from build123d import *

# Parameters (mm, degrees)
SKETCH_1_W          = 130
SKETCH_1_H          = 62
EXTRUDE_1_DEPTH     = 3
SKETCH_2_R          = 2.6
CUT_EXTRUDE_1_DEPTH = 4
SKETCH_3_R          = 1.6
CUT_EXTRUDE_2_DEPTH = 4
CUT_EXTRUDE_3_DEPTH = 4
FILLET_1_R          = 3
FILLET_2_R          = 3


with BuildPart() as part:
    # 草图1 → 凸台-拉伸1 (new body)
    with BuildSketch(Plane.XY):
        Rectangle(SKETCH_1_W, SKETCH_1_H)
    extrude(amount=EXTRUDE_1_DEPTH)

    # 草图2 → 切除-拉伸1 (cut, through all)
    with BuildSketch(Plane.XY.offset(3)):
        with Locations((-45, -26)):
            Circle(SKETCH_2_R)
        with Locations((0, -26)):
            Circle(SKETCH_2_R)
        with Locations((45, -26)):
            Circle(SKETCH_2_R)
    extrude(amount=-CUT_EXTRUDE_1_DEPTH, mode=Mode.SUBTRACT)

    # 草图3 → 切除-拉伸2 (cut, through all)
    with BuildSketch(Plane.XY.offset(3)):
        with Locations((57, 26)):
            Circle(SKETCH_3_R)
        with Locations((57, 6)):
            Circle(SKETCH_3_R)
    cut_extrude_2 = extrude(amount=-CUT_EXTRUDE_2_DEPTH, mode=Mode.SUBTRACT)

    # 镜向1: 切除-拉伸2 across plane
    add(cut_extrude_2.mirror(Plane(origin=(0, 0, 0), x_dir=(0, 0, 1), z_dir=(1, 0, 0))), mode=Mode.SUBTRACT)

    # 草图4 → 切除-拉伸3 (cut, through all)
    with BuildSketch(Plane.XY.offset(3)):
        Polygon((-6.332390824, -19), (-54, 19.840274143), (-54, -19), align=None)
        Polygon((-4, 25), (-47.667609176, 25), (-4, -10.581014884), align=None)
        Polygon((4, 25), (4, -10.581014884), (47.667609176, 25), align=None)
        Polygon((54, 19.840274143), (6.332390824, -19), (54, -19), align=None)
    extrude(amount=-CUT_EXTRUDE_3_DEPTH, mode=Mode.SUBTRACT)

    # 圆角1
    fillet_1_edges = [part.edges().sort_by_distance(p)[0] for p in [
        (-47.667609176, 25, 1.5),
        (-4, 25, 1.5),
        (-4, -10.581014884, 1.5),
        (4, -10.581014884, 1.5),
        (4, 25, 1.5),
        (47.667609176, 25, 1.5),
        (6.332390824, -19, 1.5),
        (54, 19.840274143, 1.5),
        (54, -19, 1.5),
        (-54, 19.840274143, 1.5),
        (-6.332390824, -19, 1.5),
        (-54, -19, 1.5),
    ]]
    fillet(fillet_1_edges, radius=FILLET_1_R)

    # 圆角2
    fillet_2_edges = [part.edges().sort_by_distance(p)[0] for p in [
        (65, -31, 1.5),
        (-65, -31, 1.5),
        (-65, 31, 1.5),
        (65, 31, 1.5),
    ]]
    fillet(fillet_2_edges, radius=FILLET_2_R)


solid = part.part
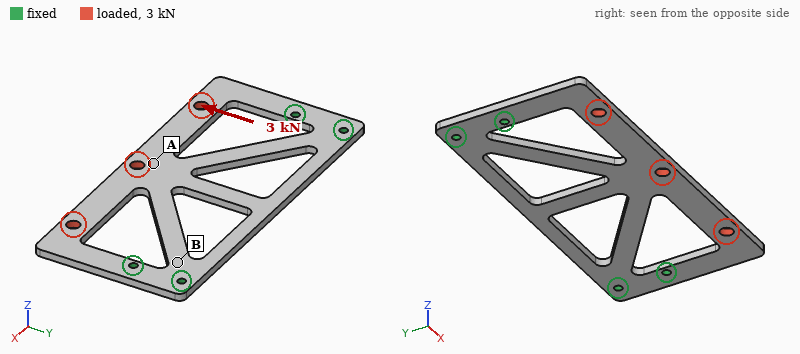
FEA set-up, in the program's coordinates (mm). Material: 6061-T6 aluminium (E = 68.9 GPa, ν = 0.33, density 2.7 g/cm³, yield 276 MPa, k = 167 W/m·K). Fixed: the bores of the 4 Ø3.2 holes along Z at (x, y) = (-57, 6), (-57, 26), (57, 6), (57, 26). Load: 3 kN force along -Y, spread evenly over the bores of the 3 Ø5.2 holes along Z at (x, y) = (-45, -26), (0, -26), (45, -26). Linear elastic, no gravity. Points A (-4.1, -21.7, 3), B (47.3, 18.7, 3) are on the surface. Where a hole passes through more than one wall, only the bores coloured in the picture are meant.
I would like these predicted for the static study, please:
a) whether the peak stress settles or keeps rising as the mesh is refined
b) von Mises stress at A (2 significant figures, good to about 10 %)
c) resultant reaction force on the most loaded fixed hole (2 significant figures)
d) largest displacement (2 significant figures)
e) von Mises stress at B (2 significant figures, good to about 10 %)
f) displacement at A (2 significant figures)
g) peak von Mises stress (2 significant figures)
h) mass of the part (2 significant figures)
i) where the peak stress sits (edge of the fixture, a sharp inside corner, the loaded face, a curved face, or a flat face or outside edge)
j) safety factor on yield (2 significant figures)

settles
20 MPa
1.0 kN
70 µm
36 MPa
63 µm
180 MPa
38 g
a curved face
1.6
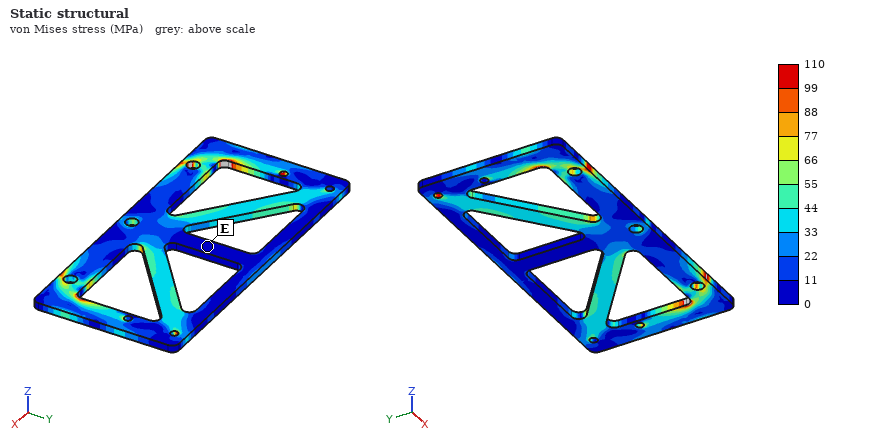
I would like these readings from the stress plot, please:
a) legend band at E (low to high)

0 to 11 MPa
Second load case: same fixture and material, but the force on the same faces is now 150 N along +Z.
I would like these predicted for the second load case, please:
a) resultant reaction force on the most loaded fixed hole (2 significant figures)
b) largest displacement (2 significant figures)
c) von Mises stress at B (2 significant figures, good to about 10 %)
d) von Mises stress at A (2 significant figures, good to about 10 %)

94 N
0.83 mm
45 MPa
33 MPa
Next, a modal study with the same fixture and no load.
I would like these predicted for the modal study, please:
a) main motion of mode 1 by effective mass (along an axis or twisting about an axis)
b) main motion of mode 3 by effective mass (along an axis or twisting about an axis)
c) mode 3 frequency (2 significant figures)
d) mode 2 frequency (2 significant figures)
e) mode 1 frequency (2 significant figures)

along Z
twisting about Y
1500 Hz
1300 Hz
630 Hz
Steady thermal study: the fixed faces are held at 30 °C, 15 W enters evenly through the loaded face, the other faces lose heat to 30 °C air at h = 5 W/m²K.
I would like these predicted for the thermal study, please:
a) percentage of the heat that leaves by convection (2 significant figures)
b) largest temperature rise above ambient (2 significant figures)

6.7 %
35 K
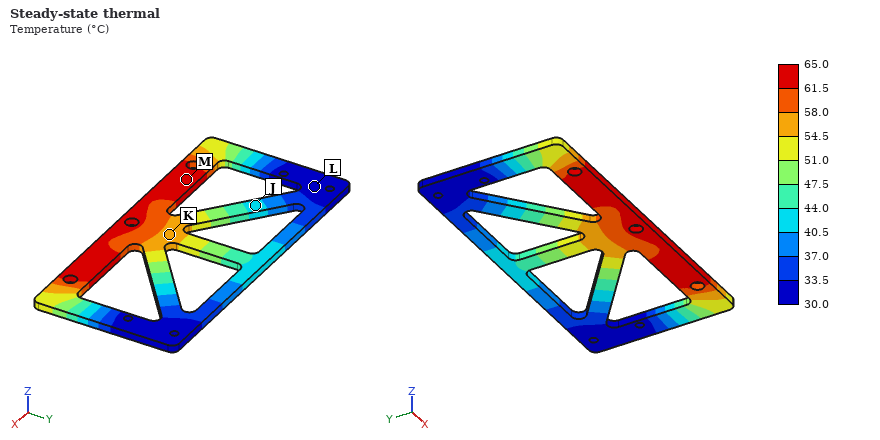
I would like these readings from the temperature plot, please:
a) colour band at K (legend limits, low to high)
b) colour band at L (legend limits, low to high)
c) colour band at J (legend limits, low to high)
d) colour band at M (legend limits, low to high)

54.5 to 58.0 °C
30.0 to 33.5 °C
40.5 to 44.0 °C
61.5 to 65.0 °C
